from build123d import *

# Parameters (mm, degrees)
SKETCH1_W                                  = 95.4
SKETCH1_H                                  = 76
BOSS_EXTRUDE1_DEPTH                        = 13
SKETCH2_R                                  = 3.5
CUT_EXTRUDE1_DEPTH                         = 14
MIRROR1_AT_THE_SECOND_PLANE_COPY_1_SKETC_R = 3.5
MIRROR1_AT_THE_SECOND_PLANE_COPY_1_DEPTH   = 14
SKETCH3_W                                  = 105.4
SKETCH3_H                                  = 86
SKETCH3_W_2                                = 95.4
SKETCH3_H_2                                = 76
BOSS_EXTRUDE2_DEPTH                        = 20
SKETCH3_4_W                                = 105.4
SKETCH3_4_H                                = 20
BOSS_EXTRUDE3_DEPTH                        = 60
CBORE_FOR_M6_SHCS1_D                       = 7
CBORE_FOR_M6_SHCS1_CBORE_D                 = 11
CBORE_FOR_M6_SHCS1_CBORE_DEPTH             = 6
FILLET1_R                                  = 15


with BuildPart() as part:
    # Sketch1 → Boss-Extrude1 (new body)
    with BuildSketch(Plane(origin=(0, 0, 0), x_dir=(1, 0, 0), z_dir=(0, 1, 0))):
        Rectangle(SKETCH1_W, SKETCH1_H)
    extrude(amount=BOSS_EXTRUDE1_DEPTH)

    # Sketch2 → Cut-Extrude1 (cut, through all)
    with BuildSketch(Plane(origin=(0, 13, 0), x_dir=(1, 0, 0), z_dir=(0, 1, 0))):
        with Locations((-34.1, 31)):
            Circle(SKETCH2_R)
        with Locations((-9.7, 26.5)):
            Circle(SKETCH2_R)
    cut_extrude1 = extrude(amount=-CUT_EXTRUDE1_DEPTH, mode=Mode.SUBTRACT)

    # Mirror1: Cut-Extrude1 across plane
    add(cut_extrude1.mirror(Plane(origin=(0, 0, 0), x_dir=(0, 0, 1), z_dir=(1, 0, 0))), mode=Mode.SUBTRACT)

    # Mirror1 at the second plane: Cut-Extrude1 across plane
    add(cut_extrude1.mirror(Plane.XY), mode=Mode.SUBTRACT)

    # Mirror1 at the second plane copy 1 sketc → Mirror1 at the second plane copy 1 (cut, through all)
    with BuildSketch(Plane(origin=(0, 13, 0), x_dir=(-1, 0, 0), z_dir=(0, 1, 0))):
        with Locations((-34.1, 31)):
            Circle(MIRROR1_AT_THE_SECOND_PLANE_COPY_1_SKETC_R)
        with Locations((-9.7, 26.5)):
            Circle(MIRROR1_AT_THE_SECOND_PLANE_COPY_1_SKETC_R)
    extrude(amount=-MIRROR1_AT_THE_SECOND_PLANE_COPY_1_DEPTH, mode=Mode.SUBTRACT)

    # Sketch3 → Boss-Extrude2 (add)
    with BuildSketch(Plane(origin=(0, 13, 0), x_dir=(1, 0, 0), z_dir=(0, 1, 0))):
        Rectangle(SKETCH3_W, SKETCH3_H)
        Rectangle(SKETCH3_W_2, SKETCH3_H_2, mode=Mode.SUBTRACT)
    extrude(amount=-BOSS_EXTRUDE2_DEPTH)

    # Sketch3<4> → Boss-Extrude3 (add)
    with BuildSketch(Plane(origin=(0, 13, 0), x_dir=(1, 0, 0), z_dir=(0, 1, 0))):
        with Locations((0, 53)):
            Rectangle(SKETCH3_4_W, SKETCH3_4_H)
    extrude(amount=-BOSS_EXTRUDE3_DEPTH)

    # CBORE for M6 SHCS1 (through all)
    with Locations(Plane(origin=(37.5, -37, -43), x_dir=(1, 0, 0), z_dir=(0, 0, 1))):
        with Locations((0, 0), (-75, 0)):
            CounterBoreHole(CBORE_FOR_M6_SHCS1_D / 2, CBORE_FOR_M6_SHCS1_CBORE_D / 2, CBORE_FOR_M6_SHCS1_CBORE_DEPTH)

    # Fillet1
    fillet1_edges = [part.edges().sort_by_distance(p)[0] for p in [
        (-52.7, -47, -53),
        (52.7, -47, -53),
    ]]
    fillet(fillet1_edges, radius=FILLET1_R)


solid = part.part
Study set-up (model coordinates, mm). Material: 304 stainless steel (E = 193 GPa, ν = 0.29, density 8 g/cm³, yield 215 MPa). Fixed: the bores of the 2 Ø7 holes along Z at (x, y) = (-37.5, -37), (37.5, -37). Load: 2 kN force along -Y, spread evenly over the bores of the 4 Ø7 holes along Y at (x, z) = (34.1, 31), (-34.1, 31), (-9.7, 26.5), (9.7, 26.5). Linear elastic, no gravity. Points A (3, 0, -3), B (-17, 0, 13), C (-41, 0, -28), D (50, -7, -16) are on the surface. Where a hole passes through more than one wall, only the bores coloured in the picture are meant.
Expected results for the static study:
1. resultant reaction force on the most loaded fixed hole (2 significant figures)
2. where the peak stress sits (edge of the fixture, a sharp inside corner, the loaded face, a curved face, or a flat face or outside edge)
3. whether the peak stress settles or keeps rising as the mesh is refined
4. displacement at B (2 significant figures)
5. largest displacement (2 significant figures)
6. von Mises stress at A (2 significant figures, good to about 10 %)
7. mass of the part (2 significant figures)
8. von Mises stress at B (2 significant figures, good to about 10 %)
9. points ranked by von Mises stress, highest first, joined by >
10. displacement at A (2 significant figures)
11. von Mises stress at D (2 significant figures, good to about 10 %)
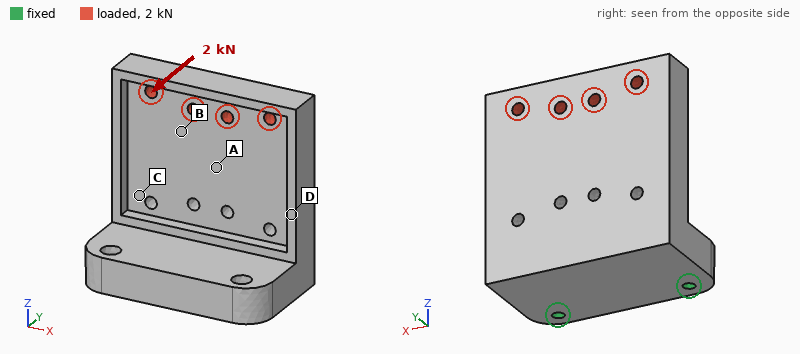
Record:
1.1 kN
edge of the fixture
keeps rising
0.099 mm
0.16 mm
16 MPa
2.0 kg
8.4 MPa
D > C > A > B
0.070 mm
42 MPa
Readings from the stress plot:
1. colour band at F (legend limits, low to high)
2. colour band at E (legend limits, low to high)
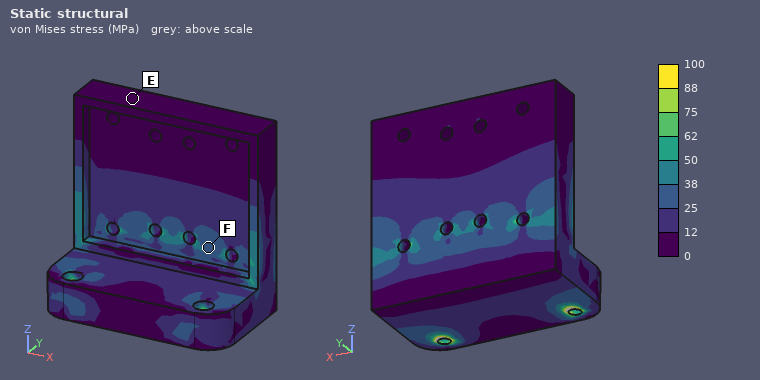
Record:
25 to 38 MPa
0 to 12 MPa
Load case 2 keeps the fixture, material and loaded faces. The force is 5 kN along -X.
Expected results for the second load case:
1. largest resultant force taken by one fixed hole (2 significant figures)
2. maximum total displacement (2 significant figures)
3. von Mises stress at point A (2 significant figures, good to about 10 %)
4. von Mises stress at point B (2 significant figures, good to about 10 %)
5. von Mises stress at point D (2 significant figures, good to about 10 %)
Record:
6.4 kN
70 µm
14 MPa
13 MPa
21 MPa
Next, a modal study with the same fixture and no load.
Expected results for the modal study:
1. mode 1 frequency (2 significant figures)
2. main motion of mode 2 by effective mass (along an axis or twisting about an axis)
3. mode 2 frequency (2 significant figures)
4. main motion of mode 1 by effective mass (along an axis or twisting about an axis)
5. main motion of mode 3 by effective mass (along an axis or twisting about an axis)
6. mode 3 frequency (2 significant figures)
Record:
840 Hz
along X
1800 Hz
along Y
along Z
2500 Hz
